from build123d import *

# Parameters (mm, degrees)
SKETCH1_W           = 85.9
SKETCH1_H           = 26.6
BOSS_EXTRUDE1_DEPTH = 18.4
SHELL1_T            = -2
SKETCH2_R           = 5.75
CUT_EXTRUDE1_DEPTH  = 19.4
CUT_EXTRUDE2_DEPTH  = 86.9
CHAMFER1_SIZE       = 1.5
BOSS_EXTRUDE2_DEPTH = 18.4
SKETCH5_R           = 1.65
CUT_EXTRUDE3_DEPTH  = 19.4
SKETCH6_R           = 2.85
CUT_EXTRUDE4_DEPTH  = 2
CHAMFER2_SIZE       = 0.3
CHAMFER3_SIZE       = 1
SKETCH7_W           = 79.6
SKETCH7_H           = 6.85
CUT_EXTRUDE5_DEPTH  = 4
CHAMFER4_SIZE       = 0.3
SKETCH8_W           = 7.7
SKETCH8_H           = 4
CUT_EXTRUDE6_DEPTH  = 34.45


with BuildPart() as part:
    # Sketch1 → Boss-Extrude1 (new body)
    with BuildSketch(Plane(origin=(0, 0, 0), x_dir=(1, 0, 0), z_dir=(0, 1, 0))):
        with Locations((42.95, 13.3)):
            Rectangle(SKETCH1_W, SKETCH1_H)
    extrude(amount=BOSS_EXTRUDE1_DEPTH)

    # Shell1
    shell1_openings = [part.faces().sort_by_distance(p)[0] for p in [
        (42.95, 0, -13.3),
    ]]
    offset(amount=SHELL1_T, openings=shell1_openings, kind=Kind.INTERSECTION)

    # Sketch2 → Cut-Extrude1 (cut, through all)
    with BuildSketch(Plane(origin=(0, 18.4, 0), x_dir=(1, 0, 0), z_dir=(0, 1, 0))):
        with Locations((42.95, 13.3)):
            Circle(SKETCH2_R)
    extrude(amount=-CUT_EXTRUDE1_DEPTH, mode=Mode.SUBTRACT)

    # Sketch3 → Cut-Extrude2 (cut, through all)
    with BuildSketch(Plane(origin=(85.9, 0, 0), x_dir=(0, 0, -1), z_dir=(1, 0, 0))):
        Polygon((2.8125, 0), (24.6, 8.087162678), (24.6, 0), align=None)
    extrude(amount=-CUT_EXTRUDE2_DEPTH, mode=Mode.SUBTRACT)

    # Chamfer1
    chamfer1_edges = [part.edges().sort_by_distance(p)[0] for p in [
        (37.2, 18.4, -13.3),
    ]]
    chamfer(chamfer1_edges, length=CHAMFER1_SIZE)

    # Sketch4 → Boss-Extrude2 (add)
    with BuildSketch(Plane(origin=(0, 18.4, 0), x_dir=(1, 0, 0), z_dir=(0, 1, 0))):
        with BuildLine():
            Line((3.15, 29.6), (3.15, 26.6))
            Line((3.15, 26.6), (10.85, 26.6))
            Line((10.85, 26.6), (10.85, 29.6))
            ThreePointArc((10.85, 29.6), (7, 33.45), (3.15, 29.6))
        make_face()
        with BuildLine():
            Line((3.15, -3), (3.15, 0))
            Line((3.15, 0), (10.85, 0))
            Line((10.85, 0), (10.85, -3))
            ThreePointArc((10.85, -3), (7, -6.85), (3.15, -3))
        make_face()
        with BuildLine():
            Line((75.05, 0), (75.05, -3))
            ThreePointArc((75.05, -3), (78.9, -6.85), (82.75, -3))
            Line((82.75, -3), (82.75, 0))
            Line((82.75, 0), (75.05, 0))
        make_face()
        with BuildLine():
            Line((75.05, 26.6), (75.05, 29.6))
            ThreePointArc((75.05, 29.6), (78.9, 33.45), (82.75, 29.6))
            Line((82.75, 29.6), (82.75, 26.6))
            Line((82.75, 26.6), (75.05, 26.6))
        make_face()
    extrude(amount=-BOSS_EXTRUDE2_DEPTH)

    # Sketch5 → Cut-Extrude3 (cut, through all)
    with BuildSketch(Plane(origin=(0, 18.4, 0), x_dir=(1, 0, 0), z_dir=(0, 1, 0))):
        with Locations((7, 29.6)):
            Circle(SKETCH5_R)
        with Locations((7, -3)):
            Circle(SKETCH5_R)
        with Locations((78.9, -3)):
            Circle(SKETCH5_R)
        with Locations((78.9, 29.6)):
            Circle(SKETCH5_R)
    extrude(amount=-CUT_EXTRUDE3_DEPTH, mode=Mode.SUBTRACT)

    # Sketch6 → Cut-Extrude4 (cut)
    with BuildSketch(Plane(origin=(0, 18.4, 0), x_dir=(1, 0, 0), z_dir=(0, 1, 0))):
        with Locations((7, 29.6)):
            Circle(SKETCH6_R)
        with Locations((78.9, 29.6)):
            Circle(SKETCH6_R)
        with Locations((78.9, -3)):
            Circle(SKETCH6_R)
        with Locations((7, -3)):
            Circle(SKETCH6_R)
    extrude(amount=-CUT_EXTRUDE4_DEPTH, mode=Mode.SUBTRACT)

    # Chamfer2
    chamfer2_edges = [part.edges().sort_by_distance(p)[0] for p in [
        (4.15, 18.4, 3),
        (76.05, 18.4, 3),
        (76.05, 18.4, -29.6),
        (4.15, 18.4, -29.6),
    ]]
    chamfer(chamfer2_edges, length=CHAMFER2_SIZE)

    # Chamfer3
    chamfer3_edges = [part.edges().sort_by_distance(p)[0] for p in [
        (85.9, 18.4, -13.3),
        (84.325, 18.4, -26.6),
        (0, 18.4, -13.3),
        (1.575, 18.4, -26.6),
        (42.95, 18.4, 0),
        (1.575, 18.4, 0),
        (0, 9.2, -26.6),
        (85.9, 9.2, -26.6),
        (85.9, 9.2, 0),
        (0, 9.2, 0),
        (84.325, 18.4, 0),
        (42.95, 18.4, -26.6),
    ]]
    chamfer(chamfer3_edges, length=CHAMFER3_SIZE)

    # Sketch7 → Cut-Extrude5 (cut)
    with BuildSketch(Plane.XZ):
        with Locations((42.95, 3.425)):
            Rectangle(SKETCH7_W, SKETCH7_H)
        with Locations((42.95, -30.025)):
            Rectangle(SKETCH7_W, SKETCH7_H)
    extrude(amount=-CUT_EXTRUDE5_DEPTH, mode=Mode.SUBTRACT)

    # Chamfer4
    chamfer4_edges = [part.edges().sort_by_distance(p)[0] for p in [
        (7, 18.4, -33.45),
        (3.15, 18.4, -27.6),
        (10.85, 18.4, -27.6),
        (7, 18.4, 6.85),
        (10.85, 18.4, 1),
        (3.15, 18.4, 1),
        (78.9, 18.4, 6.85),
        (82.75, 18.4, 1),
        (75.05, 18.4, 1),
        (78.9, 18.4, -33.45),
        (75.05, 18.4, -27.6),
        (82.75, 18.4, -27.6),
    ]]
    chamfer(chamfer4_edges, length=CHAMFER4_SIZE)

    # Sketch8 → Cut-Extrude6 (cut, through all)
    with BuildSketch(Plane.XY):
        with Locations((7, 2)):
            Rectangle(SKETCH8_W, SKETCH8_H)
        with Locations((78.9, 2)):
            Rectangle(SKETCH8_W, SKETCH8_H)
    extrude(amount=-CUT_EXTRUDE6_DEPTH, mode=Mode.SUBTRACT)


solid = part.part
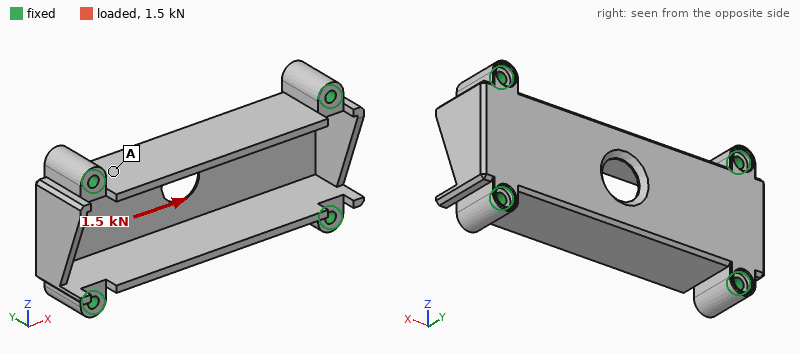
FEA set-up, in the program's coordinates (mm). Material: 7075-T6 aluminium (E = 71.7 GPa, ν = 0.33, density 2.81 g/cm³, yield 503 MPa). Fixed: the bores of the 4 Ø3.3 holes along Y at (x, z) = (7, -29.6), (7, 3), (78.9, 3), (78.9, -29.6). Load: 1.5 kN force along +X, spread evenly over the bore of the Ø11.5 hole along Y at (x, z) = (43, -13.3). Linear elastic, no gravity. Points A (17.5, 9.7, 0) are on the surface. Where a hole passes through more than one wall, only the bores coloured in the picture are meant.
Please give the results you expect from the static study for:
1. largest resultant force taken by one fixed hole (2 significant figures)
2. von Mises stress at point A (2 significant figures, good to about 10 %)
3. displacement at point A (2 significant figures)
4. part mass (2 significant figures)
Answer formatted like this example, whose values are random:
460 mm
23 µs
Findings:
380 N
9.6 MPa
2.1 µm
36 g
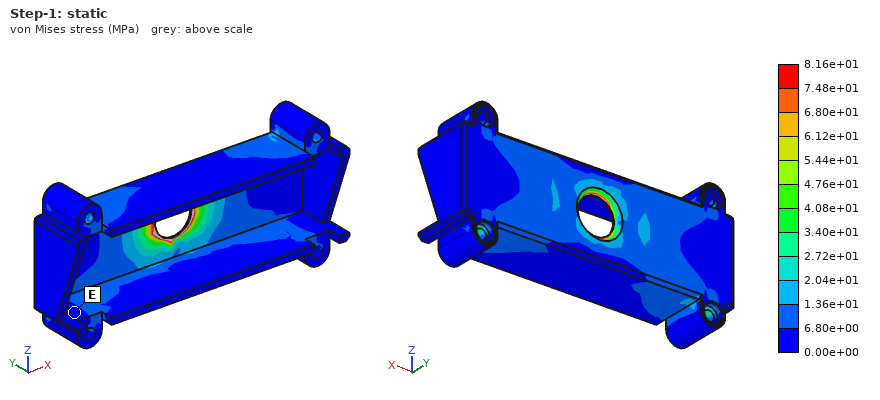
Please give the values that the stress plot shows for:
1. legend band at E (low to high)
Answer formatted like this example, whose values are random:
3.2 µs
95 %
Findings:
0.00e+00 to 6.80e+00 MPa
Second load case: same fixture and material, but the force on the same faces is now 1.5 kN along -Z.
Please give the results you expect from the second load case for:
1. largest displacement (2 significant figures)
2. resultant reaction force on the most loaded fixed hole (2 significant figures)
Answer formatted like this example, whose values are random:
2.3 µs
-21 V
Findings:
35 µm
590 N
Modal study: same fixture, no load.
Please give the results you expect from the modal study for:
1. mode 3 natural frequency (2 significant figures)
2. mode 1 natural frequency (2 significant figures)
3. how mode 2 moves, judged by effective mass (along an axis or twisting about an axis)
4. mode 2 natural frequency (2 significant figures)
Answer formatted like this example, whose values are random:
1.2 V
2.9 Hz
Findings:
8500 Hz
4400 Hz
along Z
5100 Hz
